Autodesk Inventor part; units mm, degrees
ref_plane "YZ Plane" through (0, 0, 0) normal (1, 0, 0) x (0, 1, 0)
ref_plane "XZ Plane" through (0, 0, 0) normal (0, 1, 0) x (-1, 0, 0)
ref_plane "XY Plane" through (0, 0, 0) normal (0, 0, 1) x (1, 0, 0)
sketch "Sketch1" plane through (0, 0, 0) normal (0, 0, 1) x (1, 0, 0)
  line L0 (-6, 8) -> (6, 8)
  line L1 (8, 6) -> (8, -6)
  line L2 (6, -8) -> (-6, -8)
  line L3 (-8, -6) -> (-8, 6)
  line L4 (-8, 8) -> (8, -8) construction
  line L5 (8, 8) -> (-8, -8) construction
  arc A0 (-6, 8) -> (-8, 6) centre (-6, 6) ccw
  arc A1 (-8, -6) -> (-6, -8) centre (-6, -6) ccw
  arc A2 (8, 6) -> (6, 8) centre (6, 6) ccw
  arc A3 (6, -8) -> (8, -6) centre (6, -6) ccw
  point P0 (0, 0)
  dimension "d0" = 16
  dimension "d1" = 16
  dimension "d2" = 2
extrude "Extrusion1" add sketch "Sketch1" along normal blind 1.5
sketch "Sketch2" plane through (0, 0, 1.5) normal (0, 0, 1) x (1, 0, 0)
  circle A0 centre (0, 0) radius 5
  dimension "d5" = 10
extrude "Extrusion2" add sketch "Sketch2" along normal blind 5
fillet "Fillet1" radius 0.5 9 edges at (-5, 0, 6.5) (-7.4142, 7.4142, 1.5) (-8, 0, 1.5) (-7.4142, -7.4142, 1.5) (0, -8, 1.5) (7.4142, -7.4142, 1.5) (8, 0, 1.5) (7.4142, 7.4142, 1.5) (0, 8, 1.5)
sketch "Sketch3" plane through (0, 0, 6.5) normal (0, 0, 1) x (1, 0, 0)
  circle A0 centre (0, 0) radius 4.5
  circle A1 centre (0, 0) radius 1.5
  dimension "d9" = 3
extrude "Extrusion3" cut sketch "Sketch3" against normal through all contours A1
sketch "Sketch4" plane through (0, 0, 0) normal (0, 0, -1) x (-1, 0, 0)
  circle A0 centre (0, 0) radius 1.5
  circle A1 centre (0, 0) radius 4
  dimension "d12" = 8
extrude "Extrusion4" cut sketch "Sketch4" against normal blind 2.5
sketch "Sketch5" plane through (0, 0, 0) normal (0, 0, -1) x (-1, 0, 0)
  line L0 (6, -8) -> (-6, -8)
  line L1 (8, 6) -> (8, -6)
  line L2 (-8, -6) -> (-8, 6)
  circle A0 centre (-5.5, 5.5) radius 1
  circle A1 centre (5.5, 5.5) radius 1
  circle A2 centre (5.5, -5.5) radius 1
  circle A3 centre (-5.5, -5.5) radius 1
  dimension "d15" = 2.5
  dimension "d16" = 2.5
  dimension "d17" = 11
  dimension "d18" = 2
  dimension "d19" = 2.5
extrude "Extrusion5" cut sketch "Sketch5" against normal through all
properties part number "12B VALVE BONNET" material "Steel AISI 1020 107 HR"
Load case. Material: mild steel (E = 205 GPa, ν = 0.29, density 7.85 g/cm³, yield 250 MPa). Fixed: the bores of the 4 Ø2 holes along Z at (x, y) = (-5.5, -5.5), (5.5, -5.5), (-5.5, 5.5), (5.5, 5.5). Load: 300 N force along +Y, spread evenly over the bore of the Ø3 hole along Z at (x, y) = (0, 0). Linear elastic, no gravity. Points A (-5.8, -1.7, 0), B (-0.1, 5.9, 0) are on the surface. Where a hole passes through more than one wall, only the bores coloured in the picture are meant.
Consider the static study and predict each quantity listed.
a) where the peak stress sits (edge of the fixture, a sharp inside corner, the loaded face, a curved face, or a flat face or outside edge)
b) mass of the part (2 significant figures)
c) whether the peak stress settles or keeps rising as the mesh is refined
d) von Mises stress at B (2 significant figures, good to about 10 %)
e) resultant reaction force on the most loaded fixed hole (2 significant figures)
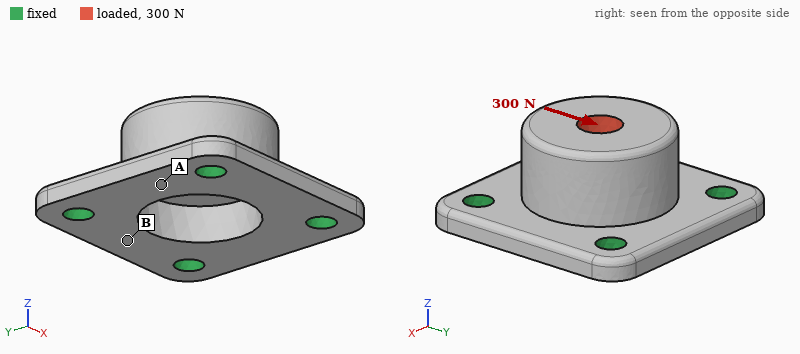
edge of the fixture
4.7 g
keeps rising
15 MPa
99 N
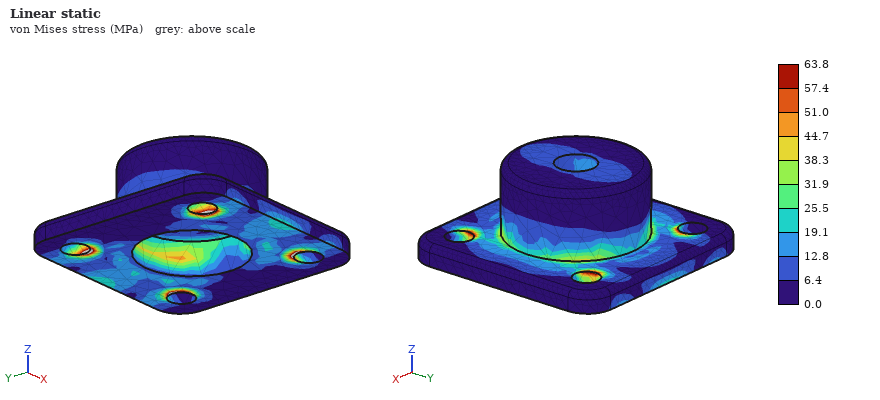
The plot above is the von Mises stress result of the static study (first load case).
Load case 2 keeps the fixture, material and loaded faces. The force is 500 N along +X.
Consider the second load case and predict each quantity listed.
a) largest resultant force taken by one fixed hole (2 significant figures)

160 N
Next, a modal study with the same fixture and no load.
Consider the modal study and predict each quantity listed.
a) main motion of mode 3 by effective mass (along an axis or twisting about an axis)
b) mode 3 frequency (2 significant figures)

along Z
46 kHz
